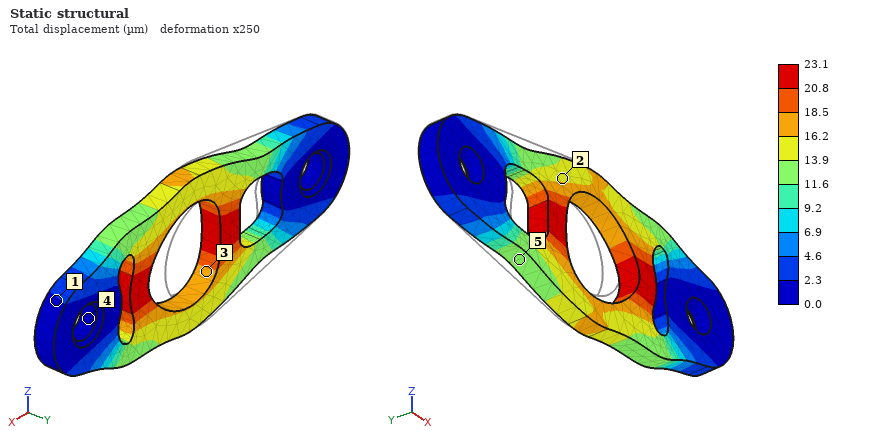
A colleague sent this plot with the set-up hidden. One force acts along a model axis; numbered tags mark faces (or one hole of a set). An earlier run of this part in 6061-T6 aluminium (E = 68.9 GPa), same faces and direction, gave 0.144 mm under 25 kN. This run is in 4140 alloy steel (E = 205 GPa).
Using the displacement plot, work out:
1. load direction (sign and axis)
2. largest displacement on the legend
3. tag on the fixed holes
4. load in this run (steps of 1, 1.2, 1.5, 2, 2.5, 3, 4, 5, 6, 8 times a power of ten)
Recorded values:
+X
23.1 µm
4
12 kN
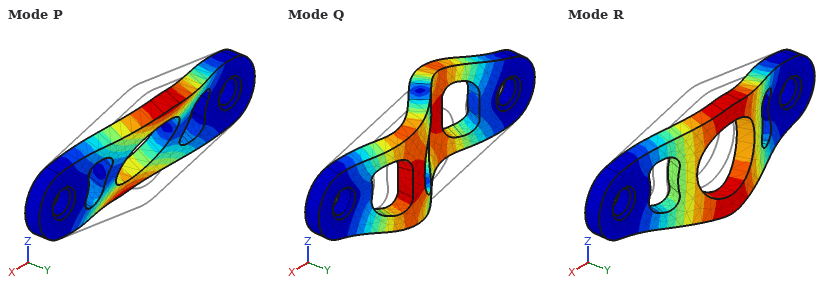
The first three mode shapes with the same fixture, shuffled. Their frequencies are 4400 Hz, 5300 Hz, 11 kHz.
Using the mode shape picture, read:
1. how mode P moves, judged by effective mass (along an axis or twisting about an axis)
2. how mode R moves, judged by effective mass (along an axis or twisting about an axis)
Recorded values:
twisting about X
along Y
